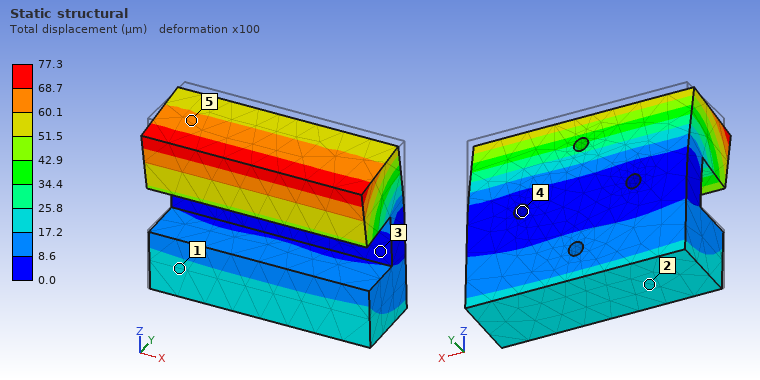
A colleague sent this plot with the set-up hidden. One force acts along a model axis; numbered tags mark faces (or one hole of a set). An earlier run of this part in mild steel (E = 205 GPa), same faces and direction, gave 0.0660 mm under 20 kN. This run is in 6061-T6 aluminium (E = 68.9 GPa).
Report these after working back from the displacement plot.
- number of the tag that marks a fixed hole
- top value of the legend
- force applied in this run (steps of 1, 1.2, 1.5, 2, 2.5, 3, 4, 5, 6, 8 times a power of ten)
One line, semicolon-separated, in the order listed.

4; 77.3 µm; 8 kN
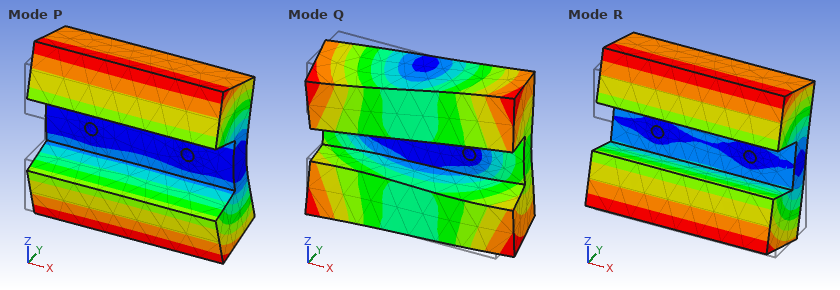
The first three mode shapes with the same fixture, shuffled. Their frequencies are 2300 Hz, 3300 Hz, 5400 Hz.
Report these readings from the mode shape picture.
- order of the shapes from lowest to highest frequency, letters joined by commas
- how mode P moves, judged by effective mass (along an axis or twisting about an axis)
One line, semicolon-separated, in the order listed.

R, P, Q; along Y
